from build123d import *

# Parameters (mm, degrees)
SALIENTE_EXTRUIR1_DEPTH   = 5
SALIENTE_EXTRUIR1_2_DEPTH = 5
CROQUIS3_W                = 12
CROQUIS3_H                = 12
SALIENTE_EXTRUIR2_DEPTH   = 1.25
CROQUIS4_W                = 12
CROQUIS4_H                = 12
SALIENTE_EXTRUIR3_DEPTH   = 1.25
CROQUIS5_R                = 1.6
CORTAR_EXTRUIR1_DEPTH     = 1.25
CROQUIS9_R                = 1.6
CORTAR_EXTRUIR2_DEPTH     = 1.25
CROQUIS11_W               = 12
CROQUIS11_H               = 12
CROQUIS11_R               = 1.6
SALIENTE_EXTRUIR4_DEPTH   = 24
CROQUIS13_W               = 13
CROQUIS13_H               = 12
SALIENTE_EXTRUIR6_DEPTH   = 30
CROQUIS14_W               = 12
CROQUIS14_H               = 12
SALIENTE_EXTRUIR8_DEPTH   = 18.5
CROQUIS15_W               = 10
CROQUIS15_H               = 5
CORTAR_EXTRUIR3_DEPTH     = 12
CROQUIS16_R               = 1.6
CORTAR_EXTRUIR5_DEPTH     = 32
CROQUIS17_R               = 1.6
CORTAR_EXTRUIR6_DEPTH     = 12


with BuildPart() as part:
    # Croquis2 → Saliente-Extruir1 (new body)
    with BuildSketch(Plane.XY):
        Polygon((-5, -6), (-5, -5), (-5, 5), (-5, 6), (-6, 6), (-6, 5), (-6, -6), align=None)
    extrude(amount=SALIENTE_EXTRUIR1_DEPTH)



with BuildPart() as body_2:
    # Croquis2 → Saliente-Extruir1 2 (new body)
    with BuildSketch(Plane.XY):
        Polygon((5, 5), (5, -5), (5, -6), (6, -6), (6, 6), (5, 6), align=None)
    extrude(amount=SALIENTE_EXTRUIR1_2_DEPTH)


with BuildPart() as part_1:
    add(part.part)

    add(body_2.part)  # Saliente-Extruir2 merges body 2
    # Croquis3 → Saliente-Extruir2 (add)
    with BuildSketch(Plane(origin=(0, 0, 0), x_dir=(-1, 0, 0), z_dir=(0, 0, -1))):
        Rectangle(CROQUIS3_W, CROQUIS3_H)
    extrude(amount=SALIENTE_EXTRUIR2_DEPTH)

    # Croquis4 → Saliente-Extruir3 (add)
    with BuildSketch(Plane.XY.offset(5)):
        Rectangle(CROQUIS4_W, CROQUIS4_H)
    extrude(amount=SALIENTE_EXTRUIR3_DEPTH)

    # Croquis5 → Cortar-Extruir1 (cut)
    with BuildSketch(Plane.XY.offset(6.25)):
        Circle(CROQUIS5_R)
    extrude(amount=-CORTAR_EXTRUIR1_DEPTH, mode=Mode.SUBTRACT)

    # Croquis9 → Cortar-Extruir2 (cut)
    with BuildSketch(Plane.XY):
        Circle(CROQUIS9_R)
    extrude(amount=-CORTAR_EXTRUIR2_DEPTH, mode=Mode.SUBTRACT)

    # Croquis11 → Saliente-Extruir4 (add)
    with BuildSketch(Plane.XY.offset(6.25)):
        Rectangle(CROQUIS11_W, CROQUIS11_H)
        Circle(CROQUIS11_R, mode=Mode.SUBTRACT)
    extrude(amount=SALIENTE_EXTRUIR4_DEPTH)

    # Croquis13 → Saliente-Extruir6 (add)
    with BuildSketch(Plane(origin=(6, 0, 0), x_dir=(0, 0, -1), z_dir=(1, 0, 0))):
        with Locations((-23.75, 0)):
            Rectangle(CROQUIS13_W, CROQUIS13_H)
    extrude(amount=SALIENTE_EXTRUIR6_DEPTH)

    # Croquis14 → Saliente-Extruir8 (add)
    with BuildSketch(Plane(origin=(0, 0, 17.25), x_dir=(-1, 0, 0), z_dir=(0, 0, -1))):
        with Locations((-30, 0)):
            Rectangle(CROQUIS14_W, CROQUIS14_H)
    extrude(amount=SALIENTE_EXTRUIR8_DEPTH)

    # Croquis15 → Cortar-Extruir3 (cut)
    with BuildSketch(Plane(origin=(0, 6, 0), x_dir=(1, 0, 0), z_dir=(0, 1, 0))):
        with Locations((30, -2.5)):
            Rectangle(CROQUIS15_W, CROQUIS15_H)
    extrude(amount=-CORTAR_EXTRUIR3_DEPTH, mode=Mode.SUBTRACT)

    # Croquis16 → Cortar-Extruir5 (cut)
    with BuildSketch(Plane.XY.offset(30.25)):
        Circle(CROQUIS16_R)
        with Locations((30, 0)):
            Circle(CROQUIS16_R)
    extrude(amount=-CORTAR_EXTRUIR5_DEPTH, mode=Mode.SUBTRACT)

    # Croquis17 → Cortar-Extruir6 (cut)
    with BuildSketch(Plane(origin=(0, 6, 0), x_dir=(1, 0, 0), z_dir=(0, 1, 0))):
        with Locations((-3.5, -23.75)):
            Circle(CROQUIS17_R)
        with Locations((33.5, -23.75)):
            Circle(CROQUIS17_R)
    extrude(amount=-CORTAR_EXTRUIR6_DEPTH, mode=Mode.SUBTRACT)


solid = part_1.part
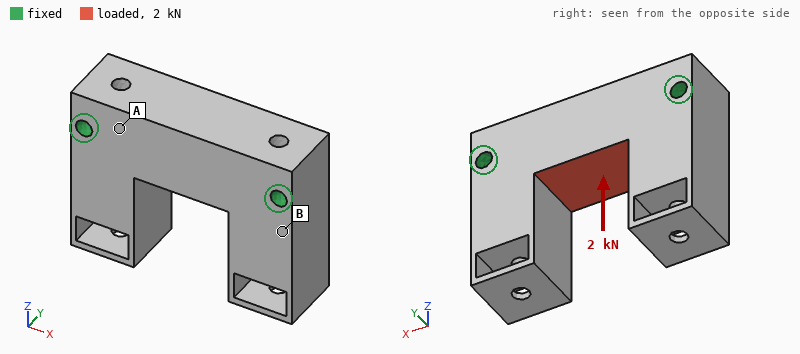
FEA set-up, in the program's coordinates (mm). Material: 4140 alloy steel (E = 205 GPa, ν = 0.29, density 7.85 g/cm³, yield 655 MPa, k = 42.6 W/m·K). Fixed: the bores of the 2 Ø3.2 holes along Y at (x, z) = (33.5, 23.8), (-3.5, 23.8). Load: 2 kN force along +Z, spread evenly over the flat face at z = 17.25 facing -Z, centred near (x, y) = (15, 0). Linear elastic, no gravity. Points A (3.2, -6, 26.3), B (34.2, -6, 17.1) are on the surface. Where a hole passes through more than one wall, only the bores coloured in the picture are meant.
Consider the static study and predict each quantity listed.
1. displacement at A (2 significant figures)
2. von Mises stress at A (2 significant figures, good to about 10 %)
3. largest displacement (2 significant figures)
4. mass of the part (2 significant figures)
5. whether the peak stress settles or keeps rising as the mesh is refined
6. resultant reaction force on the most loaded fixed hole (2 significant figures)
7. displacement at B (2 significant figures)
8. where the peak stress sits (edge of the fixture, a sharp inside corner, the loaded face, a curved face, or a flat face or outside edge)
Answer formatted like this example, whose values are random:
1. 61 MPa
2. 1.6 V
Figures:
1. 1.7 µm
2. 16 MPa
3. 6.0 µm
4. 79 g
5. keeps rising
6. 1.0 kN
7. 1.1 µm
8. edge of the fixture
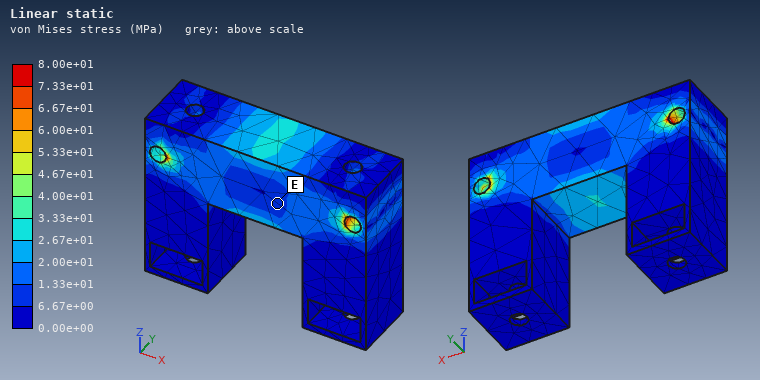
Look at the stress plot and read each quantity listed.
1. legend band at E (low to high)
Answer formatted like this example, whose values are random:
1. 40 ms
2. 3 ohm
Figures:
1. 6.67e+00 to 1.33e+01 MPa
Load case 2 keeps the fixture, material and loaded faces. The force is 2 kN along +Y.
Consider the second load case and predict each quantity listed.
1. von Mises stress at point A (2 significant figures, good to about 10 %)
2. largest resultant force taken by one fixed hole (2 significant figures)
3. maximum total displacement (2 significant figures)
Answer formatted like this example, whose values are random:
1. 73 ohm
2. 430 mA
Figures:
1. 15 MPa
2. 1.0 kN
3. 5.7 µm
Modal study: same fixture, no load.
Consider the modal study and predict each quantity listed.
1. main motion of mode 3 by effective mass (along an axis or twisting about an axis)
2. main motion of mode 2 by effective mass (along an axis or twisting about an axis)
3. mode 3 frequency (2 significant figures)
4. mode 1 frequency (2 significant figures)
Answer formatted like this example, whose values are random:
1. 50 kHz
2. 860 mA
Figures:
1. along Y
2. along X
3. 15 kHz
4. 12 kHz
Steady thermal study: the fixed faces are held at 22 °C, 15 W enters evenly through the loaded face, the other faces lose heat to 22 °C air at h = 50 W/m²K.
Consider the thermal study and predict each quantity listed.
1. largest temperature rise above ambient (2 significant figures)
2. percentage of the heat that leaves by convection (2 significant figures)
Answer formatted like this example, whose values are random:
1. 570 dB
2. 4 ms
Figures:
1. 22 K
2. 10 %
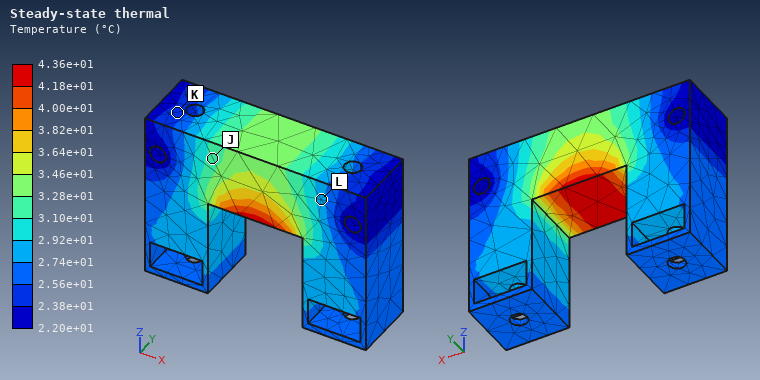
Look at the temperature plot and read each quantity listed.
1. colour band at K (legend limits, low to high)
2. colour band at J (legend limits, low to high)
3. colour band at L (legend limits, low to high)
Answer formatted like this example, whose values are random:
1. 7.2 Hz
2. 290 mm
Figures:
1. 2.38e+01 to 2.56e+01 °C
2. 3.10e+01 to 3.28e+01 °C
3. 2.74e+01 to 2.92e+01 °C
